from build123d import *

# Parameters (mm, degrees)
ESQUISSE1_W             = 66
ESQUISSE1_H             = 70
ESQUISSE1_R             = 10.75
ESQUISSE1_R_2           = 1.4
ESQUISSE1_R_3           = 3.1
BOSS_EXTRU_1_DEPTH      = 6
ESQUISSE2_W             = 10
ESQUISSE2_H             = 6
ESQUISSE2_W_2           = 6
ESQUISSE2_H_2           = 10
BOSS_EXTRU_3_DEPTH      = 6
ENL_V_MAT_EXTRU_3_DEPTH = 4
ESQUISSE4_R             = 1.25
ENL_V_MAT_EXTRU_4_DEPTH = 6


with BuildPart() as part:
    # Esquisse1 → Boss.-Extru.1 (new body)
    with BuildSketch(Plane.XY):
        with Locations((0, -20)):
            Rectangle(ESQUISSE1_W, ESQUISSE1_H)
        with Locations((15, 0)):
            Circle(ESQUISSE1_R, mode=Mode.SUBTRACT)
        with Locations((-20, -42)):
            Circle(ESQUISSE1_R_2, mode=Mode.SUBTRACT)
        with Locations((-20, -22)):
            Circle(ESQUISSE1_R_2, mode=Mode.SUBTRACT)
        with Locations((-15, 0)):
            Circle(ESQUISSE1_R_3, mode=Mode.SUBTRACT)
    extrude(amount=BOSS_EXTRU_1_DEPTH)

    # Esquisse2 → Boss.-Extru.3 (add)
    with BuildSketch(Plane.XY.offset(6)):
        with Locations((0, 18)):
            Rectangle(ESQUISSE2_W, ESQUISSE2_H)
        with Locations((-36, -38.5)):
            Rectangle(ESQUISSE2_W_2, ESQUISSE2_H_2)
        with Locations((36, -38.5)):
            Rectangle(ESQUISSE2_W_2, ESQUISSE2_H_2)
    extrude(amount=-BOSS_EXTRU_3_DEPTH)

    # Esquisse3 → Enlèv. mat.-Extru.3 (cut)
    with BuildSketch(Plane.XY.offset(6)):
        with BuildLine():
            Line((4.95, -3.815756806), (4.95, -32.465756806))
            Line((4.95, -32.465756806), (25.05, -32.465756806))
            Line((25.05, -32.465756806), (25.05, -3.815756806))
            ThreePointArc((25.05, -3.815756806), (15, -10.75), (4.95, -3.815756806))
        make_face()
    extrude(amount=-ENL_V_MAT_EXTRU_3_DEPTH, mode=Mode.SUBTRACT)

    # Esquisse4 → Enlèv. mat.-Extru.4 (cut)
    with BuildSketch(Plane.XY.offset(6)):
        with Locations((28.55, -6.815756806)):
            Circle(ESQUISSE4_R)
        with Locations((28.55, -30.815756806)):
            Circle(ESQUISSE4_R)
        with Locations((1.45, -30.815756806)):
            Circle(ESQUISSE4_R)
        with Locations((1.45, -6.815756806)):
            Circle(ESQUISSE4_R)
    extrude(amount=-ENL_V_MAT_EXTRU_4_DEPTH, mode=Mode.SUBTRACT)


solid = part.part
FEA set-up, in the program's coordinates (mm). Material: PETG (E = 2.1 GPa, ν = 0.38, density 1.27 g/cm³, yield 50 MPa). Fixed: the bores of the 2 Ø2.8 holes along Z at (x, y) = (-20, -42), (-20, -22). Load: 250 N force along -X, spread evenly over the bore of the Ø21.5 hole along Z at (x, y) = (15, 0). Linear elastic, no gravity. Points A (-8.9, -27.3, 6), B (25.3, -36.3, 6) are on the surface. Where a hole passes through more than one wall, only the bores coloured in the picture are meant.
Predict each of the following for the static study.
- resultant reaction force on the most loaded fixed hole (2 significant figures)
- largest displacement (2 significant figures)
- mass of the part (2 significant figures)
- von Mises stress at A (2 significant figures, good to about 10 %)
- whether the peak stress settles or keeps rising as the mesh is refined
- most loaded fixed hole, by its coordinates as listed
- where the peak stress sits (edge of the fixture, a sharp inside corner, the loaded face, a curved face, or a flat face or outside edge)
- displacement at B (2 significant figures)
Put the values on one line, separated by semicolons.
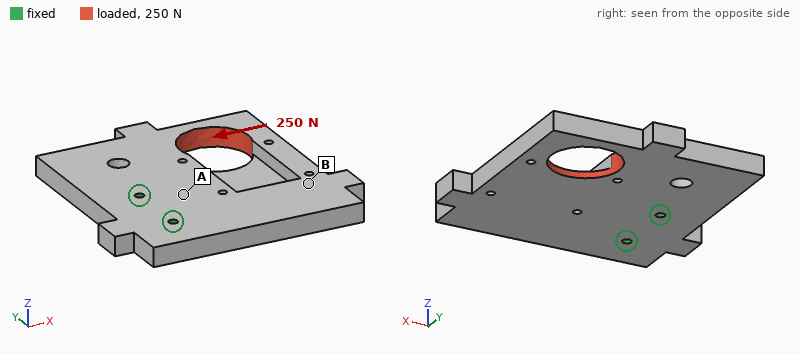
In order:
530 N; 0.32 mm; 31 g; 3.1 MPa; keeps rising; (-20, -22); edge of the fixture; 0.15 mm
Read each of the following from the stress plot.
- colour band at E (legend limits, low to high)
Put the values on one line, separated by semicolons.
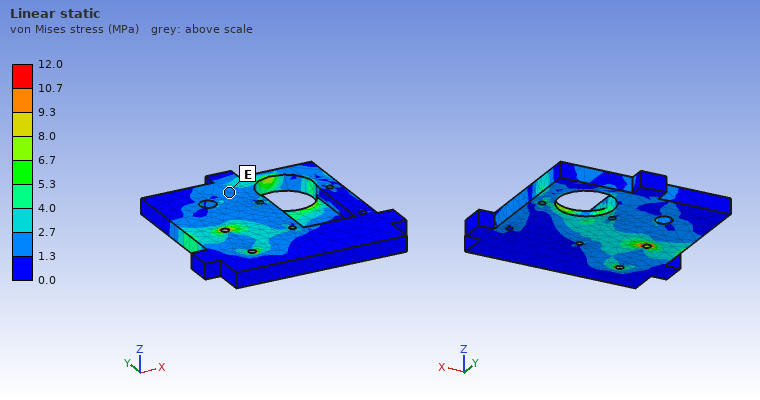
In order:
1.3 to 2.7 MPa
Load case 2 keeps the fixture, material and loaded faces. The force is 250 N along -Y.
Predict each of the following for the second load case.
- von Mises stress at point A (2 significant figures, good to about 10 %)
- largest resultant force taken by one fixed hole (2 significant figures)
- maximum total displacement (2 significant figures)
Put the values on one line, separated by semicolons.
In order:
4.0 MPa; 430 N; 0.33 mm
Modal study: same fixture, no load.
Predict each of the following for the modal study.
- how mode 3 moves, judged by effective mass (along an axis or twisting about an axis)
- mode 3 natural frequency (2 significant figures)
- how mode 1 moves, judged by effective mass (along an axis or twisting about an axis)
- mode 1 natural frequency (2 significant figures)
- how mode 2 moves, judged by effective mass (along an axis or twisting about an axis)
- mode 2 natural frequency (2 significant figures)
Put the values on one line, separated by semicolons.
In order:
along Z; 950 Hz; along Z; 360 Hz; twisting about X; 540 Hz
